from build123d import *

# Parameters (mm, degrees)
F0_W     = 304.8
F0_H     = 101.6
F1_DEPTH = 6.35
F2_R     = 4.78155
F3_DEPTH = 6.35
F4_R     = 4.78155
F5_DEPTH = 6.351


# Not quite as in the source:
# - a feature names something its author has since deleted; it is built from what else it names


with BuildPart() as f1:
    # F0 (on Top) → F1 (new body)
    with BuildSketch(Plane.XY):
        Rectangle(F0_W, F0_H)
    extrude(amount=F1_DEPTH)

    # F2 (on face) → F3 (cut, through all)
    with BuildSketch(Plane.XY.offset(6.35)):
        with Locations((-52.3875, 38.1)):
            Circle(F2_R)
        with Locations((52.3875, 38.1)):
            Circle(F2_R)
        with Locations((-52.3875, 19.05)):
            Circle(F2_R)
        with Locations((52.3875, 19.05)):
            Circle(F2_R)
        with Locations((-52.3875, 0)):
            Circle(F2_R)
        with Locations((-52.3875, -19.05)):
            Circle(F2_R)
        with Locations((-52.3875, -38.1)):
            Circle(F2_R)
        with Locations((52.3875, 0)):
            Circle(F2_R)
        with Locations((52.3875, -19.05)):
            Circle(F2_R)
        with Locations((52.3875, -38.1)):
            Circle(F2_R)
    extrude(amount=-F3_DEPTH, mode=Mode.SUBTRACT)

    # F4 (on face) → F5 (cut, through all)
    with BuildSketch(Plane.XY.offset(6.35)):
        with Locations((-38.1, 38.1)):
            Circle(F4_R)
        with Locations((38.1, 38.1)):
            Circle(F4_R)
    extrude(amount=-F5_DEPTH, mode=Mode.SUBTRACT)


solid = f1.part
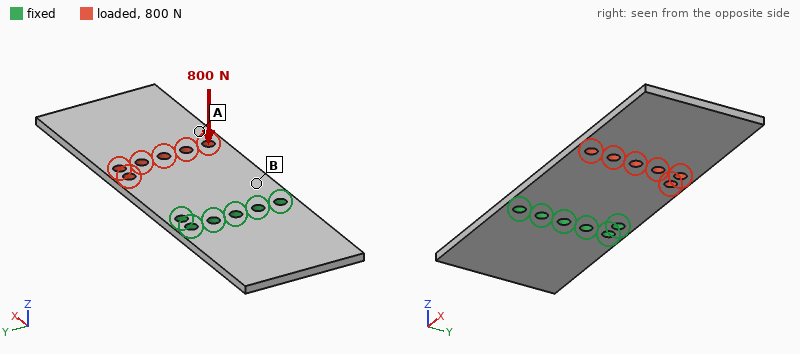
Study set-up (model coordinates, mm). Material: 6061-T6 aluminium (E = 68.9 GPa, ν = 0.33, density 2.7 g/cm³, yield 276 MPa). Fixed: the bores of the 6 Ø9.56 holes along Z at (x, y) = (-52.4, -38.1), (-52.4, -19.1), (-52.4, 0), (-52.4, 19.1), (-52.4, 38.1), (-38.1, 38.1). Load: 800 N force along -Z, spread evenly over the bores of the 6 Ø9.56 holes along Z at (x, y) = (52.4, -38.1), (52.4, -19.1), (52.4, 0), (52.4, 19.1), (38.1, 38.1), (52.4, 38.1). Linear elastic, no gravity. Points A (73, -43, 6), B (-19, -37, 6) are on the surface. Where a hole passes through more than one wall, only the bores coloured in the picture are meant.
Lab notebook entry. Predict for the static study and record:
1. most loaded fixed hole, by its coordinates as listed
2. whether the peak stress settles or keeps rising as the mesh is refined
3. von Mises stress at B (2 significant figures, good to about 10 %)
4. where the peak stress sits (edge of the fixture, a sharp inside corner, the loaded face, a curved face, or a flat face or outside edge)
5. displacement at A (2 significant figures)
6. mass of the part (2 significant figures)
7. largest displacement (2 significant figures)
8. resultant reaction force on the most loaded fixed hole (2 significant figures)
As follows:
(-38.1, 38.1)
keeps rising
65 MPa
edge of the fixture
1.9 mm
520 g
3.7 mm
1.1 kN
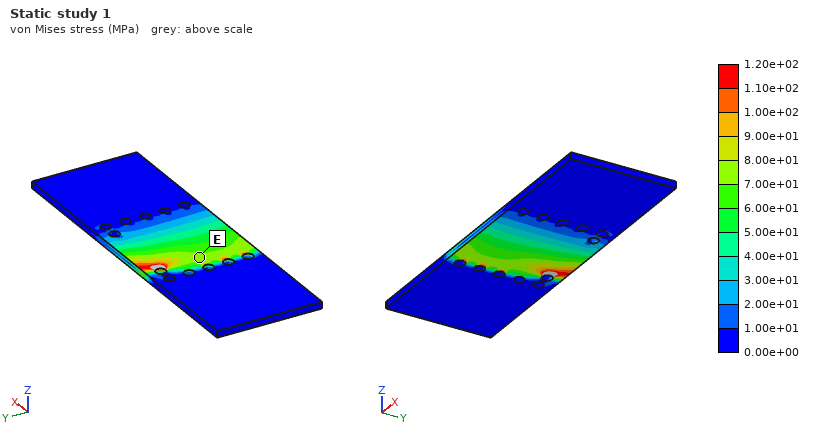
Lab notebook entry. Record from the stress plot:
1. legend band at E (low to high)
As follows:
7.00e+01 to 8.00e+01 MPa
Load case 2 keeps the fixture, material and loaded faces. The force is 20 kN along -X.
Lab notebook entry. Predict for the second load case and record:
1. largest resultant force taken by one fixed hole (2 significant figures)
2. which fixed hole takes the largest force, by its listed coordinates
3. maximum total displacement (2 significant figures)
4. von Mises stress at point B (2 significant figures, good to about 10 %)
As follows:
6.2 kN
(-38.1, 38.1)
65 µm
23 MPa
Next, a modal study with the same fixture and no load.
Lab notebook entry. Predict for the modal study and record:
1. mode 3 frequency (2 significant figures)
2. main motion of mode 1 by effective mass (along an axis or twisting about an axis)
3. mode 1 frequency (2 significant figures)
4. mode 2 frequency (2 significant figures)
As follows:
570 Hz
along Z
140 Hz
550 Hz
